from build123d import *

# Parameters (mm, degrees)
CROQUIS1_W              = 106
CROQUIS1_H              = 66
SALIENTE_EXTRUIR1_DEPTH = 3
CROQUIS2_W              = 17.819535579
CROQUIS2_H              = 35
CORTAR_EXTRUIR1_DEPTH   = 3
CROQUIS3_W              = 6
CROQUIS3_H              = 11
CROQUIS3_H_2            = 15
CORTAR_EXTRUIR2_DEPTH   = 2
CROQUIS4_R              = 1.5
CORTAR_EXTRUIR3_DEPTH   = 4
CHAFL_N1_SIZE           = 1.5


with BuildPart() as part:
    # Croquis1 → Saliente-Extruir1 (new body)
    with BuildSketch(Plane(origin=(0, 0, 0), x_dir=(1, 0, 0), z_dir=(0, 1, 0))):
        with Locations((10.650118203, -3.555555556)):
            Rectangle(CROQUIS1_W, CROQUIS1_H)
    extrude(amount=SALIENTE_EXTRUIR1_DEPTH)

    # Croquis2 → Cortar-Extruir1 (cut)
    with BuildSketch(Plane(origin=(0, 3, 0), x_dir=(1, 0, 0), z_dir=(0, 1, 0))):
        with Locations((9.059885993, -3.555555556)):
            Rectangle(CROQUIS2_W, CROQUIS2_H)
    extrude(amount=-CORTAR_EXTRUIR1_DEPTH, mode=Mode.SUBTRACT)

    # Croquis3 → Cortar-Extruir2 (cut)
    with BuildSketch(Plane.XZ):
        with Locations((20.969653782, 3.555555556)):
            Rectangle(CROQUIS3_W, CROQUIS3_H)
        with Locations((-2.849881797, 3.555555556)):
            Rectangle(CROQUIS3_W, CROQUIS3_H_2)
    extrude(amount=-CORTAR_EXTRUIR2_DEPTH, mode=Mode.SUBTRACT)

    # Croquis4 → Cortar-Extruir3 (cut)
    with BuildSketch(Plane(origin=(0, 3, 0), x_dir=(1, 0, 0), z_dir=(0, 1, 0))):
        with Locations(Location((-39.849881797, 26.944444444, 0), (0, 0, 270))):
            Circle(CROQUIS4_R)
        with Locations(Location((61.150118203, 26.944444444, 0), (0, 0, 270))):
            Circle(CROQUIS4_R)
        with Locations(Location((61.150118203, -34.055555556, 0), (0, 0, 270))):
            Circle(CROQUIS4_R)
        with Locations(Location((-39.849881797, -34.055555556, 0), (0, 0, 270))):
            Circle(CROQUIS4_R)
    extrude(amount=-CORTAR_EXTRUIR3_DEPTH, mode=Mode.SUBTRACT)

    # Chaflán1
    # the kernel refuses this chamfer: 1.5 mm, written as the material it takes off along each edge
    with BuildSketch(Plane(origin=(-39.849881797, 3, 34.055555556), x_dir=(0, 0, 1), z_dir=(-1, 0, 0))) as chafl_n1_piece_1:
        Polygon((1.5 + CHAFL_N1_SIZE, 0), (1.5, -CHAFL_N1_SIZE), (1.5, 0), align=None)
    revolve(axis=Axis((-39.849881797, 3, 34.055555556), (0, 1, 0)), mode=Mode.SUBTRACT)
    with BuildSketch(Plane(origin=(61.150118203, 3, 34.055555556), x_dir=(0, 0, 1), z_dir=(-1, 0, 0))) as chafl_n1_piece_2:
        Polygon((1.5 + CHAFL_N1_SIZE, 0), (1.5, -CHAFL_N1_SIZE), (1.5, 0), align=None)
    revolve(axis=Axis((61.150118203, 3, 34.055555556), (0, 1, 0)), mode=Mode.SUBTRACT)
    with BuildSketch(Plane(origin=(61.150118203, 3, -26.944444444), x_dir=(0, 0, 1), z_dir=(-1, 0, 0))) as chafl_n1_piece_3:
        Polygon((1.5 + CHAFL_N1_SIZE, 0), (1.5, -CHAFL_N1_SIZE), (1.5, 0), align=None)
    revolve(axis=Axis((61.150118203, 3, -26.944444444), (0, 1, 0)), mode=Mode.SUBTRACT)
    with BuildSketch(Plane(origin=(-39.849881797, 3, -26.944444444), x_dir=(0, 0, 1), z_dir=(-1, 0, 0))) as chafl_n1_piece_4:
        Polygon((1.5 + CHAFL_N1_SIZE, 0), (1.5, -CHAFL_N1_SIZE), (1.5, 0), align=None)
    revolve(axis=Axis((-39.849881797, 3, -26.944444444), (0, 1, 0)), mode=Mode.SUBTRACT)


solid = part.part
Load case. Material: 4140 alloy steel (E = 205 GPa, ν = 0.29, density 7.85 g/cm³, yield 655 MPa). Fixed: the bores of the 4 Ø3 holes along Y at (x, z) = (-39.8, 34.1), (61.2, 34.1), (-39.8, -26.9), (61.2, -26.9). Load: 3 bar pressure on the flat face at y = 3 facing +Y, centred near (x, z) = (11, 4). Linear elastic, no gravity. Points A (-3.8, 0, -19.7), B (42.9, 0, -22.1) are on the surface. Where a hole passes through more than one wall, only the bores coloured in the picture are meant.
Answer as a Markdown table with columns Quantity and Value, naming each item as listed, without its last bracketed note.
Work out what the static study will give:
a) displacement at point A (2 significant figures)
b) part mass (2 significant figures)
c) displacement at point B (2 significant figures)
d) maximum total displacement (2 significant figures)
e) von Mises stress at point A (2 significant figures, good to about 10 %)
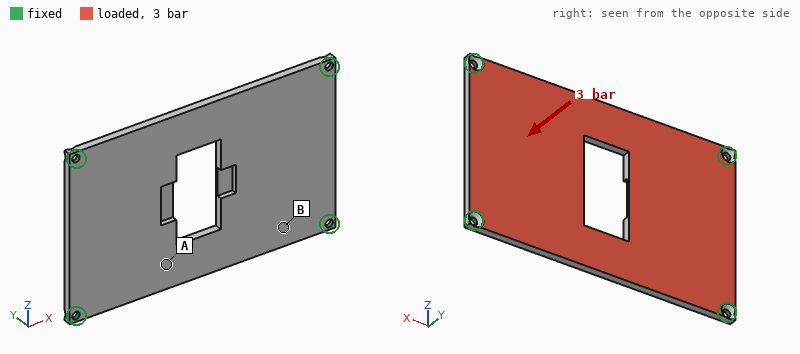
| Quantity | Value |
|---|---|
| displacement at point A | 0.39 mm |
| part mass | 150 g |
| displacement at point B | 0.20 mm |
| maximum total displacement | 0.51 mm |
| von Mises stress at point A | 120 MPa |
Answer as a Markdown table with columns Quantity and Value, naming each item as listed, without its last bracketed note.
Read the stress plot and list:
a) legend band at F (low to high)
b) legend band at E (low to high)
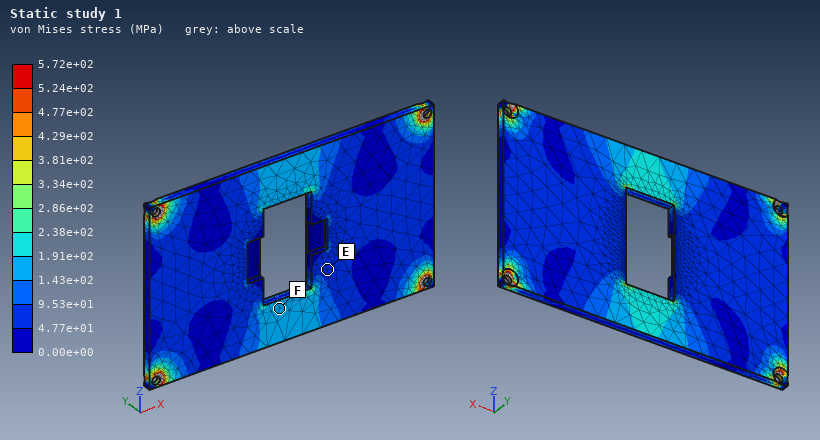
| Quantity | Value |
|---|---|
| legend band at F | 1.43e+02 to 1.91e+02 MPa |
| legend band at E | 4.77e+01 to 9.53e+01 MPa |
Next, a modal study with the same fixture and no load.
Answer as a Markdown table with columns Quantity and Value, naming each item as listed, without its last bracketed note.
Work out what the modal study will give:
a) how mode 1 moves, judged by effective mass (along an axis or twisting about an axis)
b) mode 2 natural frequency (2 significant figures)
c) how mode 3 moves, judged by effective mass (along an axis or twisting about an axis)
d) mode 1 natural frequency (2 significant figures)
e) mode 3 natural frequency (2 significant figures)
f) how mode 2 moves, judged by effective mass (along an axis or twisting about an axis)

| Quantity | Value |
|---|---|
| how mode 1 moves, judged by effective mass | along Y |
| mode 2 natural frequency | 1900 Hz |
| how mode 3 moves, judged by effective mass | twisting about Z |
| mode 1 natural frequency | 1000 Hz |
| mode 3 natural frequency | 2500 Hz |
| how mode 2 moves, judged by effective mass | twisting about X |
